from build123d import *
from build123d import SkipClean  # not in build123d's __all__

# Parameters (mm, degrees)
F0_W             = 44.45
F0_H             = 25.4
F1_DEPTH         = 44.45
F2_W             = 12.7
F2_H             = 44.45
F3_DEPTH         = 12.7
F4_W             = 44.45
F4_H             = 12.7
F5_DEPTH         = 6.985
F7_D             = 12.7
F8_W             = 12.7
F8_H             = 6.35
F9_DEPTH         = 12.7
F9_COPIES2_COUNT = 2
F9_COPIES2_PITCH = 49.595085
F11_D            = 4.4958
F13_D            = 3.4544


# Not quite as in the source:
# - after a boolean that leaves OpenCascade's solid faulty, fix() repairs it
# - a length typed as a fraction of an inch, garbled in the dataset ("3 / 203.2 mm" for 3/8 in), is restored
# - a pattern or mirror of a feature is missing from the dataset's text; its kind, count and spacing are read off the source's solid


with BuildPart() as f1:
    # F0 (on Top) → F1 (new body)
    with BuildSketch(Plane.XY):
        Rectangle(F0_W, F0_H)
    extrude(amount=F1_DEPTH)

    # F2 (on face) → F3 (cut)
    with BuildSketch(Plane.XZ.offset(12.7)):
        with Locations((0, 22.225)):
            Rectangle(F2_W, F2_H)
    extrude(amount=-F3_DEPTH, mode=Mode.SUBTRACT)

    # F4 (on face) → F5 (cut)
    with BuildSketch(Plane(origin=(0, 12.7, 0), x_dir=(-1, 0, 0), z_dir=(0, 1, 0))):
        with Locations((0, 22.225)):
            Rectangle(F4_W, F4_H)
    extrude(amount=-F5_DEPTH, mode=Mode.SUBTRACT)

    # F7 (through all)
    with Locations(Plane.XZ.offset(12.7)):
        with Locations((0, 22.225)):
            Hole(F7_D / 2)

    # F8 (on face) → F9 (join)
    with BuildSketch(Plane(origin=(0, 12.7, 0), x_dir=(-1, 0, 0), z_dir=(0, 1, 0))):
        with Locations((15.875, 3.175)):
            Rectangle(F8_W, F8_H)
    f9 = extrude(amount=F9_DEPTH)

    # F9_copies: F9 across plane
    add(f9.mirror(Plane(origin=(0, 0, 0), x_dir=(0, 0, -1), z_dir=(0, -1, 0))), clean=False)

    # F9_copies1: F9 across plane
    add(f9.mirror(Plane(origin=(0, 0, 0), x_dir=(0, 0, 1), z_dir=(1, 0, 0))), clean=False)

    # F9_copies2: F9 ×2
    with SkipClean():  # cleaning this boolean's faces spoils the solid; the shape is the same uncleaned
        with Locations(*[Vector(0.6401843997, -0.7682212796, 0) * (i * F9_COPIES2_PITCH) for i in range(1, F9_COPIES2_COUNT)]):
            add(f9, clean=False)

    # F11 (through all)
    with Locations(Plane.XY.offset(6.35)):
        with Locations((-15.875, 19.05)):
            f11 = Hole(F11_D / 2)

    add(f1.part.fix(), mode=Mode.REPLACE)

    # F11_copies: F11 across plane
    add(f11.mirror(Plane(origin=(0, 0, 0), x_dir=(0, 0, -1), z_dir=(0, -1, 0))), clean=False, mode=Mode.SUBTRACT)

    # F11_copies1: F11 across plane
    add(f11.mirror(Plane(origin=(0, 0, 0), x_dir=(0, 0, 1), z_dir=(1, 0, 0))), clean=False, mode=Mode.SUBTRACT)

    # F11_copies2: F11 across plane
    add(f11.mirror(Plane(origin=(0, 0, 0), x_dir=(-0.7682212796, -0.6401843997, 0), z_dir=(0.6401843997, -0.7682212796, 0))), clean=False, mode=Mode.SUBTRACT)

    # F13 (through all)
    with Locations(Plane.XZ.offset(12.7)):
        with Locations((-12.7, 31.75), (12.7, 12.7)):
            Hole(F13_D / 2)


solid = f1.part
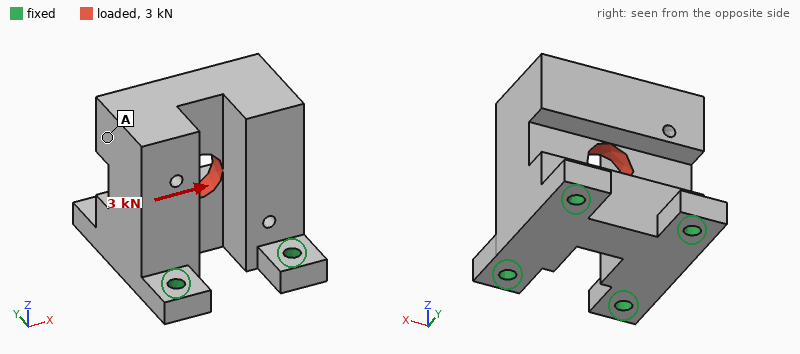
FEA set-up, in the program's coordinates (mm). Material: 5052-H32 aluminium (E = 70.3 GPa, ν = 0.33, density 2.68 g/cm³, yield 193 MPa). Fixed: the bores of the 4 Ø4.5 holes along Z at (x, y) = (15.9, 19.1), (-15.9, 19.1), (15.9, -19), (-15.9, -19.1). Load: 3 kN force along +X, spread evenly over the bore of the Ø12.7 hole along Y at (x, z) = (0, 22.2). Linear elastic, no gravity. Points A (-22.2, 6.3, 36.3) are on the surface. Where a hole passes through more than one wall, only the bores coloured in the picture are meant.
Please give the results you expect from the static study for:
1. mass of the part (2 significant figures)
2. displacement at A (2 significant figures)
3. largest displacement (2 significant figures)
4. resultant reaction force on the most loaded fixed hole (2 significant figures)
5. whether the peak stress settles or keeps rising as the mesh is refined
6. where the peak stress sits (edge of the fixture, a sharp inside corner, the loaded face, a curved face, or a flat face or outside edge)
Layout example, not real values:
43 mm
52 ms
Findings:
110 g
28 µm
33 µm
1.4 kN
keeps rising
edge of the fixture
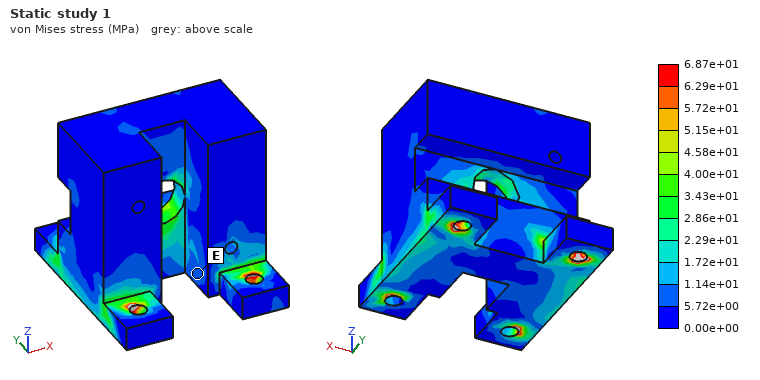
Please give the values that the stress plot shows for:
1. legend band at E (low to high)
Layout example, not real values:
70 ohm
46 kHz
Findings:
5.72e+00 to 1.14e+01 MPa
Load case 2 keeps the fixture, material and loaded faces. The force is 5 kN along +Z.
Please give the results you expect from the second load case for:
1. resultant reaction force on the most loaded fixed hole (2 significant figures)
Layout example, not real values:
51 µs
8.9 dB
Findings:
1.6 kN
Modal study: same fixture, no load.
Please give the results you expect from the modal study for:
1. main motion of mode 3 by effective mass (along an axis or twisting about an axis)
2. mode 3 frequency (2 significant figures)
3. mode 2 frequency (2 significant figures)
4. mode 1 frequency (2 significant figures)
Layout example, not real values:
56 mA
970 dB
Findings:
twisting about Z
9300 Hz
5600 Hz
5400 Hz
